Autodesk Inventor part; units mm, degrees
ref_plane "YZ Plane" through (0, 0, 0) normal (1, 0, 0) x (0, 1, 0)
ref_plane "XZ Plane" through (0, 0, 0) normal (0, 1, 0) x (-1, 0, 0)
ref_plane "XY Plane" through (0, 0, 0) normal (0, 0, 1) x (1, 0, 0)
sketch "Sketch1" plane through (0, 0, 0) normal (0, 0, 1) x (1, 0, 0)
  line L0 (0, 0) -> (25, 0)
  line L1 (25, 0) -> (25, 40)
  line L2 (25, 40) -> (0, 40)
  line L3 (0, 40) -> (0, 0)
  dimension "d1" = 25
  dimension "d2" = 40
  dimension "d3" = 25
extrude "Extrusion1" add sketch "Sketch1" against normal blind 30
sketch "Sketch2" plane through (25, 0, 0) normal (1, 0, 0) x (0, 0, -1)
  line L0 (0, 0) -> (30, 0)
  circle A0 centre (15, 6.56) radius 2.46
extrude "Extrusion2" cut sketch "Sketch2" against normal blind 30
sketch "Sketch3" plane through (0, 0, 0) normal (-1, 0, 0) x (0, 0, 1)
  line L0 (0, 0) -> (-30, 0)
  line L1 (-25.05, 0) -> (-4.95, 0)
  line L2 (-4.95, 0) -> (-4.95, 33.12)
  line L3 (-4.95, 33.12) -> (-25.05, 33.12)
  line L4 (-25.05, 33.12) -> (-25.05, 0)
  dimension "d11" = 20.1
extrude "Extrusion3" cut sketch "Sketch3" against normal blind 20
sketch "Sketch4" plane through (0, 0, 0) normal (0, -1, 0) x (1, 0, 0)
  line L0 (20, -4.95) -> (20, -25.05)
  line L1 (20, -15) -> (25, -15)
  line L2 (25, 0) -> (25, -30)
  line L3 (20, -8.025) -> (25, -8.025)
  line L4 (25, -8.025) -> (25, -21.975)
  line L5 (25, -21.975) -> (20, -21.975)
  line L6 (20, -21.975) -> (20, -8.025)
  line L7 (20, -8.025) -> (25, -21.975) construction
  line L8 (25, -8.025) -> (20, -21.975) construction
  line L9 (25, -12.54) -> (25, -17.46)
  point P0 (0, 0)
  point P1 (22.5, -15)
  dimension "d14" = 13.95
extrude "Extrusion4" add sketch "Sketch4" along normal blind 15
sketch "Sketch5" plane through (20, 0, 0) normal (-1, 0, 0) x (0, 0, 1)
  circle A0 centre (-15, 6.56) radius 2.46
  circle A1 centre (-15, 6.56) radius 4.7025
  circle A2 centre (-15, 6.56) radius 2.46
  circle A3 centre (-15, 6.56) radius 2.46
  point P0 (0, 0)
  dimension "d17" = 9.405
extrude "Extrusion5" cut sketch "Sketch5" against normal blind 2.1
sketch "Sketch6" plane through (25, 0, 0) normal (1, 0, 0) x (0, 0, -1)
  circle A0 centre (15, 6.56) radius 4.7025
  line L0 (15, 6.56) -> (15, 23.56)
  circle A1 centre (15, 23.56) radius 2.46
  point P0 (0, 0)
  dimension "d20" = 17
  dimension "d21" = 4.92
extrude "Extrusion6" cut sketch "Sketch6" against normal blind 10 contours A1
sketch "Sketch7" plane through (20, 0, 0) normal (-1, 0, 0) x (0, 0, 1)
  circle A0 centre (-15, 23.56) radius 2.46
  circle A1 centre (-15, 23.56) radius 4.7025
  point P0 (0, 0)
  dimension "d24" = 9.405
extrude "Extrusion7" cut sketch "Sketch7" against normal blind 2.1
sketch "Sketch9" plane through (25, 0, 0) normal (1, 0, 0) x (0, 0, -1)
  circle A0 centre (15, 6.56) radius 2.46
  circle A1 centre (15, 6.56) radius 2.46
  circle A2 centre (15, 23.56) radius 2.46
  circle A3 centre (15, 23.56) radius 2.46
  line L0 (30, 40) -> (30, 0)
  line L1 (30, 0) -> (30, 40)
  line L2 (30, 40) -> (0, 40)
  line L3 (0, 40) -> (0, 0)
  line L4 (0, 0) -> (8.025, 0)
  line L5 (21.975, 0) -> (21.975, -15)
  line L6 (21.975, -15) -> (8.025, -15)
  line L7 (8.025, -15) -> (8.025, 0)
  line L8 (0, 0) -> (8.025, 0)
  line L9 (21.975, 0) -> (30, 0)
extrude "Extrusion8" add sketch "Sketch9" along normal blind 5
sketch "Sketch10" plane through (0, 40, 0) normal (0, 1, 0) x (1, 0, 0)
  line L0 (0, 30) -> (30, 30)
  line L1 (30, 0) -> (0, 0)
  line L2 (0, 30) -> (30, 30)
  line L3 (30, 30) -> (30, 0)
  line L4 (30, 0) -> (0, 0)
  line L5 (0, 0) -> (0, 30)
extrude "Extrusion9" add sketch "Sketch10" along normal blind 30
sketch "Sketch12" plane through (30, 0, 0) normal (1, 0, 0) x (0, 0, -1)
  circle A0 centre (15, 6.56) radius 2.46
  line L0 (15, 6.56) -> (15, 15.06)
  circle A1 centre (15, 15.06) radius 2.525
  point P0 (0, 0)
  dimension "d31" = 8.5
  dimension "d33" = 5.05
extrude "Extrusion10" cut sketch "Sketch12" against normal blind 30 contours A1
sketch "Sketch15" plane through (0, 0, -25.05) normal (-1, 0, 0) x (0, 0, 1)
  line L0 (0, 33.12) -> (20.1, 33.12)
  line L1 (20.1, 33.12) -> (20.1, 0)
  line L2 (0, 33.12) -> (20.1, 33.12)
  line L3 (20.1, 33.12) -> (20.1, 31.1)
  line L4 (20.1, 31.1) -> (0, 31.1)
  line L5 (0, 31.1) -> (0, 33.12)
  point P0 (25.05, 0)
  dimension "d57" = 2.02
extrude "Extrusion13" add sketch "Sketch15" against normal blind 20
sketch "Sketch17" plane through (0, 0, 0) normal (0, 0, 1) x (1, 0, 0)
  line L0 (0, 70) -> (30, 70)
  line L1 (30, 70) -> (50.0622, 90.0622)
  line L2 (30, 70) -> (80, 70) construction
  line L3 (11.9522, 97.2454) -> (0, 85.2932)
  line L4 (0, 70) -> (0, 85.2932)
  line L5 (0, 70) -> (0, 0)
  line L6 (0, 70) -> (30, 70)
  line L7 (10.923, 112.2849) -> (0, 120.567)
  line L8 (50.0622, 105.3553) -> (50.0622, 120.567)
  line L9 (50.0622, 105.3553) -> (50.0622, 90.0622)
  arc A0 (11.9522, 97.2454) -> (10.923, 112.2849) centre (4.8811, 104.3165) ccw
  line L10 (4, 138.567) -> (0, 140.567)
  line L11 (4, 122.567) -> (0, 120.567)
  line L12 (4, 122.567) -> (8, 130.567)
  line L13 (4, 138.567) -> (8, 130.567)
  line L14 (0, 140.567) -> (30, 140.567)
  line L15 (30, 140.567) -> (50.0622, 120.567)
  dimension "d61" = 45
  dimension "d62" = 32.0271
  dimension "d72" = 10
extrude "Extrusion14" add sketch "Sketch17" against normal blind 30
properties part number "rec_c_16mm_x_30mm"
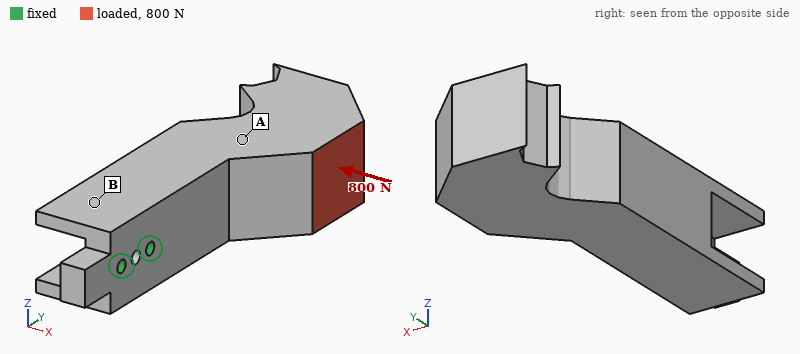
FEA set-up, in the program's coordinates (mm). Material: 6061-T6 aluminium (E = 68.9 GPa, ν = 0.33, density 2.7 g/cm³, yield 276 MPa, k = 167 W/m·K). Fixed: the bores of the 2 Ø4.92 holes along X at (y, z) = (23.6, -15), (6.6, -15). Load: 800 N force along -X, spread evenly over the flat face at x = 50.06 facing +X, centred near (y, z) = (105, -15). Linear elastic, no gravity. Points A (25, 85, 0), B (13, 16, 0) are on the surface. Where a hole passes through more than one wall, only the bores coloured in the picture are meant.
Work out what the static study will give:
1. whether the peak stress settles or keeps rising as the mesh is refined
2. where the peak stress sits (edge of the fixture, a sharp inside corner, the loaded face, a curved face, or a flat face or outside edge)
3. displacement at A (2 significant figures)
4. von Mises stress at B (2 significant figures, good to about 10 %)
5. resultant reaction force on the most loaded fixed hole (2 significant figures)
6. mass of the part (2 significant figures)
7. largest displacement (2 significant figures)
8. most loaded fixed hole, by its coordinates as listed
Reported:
keeps rising
edge of the fixture
0.11 mm
18 MPa
3.4 kN
360 g
0.22 mm
(23.6, -15)
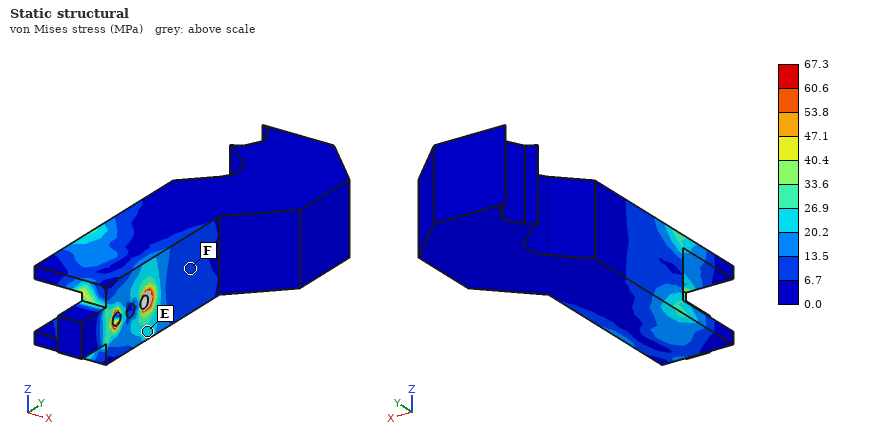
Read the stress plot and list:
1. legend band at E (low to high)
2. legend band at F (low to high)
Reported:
20.2 to 26.9 MPa
6.7 to 13.5 MPa
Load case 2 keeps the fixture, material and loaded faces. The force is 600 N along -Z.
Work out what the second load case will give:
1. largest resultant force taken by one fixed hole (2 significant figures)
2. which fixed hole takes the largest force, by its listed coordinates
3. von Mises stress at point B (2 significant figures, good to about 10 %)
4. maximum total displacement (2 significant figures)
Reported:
2.7 kN
(23.6, -15)
9.7 MPa
0.15 mm
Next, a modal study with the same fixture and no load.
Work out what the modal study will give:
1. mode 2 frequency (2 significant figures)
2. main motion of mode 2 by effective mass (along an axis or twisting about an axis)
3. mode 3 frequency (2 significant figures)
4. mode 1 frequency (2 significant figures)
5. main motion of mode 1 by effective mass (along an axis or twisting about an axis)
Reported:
860 Hz
along Z
2400 Hz
750 Hz
along X
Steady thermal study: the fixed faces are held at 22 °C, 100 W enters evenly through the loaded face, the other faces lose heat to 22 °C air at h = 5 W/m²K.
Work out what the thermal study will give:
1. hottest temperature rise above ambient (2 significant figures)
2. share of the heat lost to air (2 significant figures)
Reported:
77 K
4.6 %
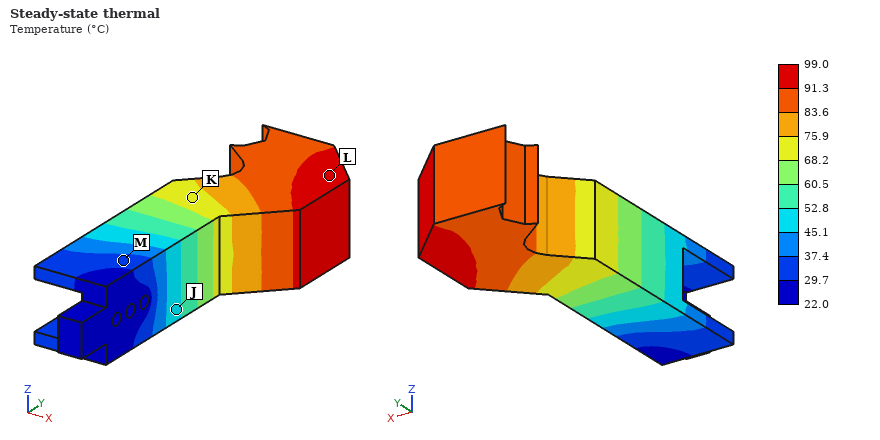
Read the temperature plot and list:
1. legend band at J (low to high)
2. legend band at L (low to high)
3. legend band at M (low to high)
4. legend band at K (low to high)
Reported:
45.1 to 52.8 °C
91.3 to 99.0 °C
29.7 to 37.4 °C
68.2 to 75.9 °C
